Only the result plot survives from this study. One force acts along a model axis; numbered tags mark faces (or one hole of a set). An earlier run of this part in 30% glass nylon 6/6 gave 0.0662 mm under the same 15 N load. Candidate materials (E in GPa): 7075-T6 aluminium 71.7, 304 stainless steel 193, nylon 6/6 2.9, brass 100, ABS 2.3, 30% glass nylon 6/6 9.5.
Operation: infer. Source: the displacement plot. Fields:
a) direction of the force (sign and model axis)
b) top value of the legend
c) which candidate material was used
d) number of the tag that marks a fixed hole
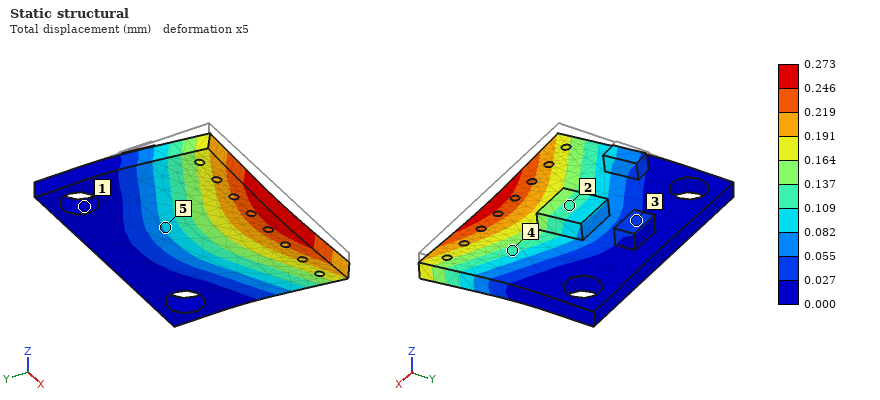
-Z
0.273 mm
ABS
1
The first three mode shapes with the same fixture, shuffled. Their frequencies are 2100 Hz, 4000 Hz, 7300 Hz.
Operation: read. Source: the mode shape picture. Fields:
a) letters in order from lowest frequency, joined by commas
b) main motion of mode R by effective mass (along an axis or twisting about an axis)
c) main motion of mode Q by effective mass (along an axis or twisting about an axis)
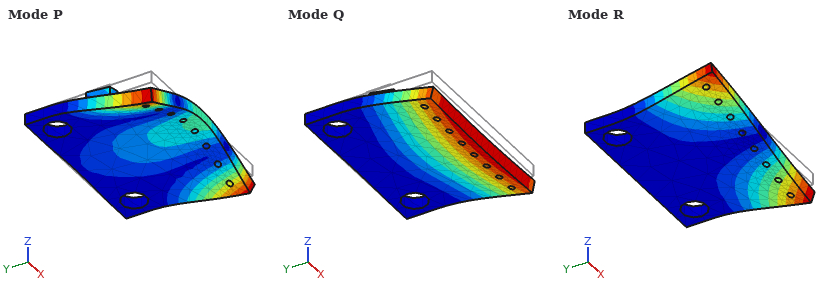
Q, R, P
twisting about Y
along Z
